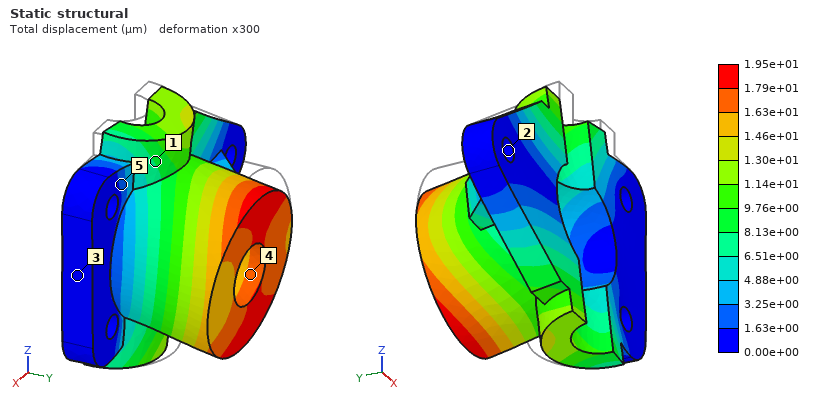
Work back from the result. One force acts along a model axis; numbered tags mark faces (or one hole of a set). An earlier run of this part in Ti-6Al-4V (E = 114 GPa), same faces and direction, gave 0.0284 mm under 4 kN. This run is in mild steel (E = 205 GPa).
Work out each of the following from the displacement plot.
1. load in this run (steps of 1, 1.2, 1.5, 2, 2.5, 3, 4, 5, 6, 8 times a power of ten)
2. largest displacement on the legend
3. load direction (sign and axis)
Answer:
5 kN
1.95e+01 µm
-Z
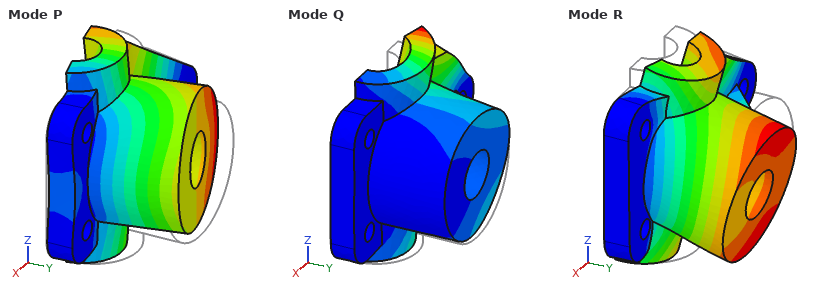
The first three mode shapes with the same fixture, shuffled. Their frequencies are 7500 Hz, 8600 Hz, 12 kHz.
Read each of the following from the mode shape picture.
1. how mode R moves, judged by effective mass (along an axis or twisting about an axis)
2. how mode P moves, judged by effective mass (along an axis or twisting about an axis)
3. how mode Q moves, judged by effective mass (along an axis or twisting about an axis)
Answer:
along Z
along Y
along Z
